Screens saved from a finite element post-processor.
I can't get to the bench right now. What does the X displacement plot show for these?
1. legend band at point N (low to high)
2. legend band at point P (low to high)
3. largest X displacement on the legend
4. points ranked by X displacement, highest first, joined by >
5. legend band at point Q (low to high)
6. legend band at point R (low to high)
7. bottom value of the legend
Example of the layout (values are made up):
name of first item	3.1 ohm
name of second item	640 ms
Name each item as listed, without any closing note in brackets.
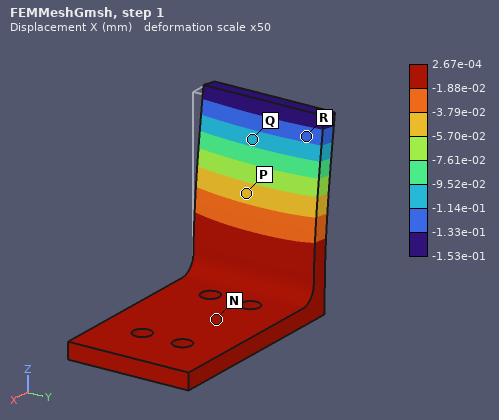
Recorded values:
legend band at point N	-1.88e-02 to 2.67e-04 mm
legend band at point P	-5.70e-02 to -3.79e-02 mm
largest X displacement on the legend	2.67e-04 mm
points ranked by X displacement, highest first, joined by >	N > P > Q > R
legend band at point Q	-1.14e-01 to -9.52e-02 mm
legend band at point R	-1.33e-01 to -1.14e-01 mm
bottom value of the legend	-1.53e-01 mm
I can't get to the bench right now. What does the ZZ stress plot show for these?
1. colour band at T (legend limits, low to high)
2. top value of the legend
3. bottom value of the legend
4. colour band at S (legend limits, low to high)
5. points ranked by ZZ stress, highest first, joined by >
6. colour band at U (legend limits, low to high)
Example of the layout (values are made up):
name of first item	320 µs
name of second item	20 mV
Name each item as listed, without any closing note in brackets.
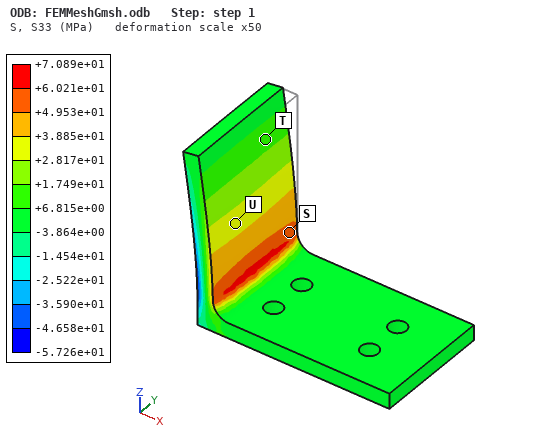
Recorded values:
colour band at T	+6.815e+00 to +1.749e+01 MPa
top value of the legend	+7.089e+01 MPa
bottom value of the legend	-5.726e+01 MPa
colour band at S	+4.953e+01 to +6.021e+01 MPa
points ranked by ZZ stress, highest first, joined by >	S > U > T
colour band at U	+2.817e+01 to +3.885e+01 MPa
